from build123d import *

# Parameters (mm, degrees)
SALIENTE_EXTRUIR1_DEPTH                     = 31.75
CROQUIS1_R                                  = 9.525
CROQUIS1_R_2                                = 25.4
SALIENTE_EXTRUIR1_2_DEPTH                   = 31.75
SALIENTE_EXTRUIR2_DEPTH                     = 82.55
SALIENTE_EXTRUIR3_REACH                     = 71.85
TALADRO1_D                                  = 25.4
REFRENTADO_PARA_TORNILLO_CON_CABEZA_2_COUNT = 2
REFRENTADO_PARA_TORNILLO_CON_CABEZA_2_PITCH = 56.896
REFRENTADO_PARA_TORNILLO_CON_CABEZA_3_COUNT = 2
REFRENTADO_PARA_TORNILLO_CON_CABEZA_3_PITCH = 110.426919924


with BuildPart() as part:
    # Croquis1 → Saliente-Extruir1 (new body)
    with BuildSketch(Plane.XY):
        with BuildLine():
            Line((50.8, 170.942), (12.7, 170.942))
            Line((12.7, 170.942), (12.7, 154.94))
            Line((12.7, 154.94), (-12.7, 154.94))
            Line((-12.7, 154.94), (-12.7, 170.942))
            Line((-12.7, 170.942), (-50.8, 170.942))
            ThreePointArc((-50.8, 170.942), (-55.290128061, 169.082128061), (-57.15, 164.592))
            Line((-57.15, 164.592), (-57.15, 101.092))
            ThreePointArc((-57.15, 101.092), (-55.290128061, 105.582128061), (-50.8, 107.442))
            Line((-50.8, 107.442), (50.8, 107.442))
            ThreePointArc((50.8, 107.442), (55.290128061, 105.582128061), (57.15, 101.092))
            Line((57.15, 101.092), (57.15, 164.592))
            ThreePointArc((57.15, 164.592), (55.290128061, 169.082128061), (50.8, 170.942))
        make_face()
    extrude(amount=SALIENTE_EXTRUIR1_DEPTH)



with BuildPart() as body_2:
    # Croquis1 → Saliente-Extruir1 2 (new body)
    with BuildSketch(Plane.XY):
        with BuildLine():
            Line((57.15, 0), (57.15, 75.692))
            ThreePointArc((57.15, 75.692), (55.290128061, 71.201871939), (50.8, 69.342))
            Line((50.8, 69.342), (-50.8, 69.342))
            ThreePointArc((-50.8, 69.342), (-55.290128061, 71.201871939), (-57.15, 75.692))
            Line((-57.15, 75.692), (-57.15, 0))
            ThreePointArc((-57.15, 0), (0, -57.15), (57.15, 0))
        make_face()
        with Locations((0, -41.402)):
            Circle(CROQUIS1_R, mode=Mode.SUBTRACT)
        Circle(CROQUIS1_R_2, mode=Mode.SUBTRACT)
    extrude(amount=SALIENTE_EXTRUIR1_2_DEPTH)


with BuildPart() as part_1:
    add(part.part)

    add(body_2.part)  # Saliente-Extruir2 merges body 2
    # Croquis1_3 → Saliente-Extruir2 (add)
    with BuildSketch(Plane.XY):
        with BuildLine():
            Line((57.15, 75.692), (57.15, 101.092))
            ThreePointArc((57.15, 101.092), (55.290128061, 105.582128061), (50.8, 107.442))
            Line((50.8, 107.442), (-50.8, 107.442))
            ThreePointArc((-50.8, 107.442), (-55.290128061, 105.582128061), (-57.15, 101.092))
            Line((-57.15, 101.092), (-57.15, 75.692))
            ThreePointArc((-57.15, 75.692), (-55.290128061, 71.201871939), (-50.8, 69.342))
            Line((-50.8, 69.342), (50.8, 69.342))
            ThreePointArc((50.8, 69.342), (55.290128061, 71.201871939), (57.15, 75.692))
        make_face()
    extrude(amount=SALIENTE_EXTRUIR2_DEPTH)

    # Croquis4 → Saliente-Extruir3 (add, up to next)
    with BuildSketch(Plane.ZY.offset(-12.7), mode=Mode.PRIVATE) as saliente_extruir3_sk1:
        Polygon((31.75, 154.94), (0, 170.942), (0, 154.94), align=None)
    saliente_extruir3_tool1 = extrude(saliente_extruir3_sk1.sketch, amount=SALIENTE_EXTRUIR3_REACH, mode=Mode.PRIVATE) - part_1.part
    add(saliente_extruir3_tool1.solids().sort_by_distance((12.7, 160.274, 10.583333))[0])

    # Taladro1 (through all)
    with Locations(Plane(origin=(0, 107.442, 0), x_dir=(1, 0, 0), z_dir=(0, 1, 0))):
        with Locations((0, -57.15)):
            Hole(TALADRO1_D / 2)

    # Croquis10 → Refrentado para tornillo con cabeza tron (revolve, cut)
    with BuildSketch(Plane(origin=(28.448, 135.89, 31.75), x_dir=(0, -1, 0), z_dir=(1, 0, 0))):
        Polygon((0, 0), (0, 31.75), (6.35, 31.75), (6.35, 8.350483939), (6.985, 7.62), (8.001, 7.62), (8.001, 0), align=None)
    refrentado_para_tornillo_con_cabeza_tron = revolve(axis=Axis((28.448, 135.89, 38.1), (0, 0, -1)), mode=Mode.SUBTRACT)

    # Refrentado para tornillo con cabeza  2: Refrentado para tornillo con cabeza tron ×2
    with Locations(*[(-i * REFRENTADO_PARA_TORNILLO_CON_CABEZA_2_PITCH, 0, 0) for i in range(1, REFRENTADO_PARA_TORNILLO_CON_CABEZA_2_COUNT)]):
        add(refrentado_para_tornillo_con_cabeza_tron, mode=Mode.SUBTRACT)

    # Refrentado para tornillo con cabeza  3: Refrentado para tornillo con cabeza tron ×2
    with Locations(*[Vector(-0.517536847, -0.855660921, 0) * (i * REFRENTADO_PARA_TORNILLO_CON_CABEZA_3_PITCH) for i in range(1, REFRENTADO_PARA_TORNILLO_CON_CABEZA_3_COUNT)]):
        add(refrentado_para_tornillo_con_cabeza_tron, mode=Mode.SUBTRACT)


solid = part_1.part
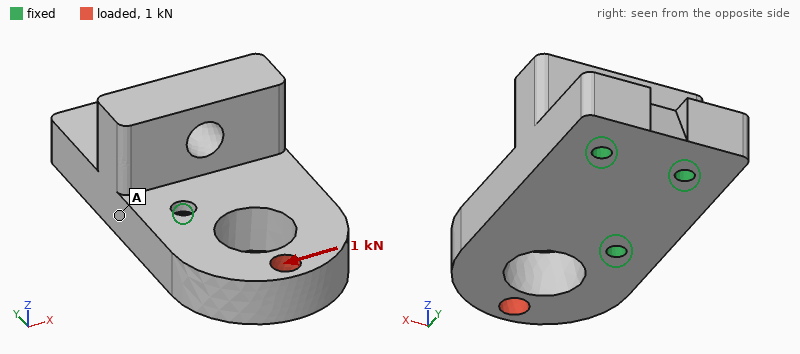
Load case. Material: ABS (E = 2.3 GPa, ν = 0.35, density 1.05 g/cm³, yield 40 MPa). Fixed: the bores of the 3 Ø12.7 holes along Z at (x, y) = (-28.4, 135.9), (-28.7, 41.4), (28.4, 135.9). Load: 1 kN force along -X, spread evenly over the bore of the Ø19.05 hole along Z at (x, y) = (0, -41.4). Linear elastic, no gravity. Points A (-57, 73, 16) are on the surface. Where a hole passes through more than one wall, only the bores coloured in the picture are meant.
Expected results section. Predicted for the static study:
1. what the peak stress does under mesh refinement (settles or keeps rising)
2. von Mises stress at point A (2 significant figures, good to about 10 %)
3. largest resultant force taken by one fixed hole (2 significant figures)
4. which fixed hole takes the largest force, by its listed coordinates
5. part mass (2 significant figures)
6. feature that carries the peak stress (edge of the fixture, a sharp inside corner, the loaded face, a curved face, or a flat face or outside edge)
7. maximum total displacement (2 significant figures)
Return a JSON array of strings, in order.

["keeps rising", "0.58 MPa", "1.5 kN", "(-28.7, 41.4)", "930 g", "edge of the fixture", "0.21 mm"]
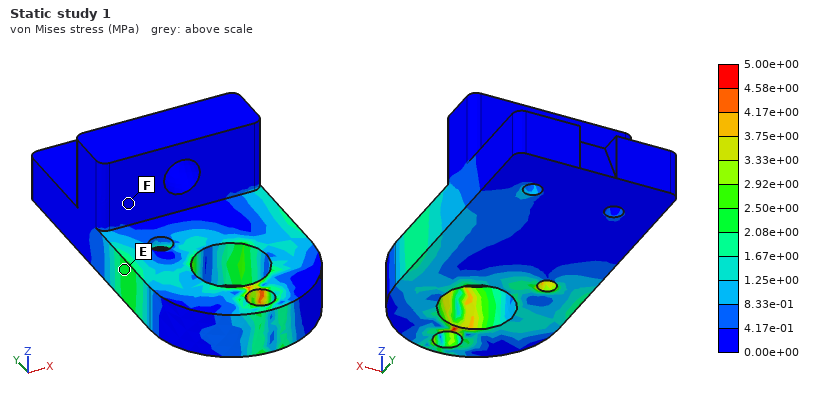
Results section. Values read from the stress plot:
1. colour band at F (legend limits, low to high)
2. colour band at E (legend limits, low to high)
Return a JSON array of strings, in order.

["0.00e+00 to 4.17e-01 MPa", "2.08e+00 to 2.50e+00 MPa"]
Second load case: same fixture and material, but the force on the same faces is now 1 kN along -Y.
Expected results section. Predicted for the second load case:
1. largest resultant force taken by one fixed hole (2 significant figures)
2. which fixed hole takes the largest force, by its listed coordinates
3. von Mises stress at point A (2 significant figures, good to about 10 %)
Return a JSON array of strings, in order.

["530 N", "(-28.7, 41.4)", "0.18 MPa"]
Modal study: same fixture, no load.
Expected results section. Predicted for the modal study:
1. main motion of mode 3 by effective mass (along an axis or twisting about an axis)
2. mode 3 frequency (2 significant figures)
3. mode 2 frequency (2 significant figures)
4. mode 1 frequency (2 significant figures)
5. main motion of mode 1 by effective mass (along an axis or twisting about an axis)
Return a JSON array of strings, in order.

["along X", "1100 Hz", "910 Hz", "550 Hz", "along Z"]
